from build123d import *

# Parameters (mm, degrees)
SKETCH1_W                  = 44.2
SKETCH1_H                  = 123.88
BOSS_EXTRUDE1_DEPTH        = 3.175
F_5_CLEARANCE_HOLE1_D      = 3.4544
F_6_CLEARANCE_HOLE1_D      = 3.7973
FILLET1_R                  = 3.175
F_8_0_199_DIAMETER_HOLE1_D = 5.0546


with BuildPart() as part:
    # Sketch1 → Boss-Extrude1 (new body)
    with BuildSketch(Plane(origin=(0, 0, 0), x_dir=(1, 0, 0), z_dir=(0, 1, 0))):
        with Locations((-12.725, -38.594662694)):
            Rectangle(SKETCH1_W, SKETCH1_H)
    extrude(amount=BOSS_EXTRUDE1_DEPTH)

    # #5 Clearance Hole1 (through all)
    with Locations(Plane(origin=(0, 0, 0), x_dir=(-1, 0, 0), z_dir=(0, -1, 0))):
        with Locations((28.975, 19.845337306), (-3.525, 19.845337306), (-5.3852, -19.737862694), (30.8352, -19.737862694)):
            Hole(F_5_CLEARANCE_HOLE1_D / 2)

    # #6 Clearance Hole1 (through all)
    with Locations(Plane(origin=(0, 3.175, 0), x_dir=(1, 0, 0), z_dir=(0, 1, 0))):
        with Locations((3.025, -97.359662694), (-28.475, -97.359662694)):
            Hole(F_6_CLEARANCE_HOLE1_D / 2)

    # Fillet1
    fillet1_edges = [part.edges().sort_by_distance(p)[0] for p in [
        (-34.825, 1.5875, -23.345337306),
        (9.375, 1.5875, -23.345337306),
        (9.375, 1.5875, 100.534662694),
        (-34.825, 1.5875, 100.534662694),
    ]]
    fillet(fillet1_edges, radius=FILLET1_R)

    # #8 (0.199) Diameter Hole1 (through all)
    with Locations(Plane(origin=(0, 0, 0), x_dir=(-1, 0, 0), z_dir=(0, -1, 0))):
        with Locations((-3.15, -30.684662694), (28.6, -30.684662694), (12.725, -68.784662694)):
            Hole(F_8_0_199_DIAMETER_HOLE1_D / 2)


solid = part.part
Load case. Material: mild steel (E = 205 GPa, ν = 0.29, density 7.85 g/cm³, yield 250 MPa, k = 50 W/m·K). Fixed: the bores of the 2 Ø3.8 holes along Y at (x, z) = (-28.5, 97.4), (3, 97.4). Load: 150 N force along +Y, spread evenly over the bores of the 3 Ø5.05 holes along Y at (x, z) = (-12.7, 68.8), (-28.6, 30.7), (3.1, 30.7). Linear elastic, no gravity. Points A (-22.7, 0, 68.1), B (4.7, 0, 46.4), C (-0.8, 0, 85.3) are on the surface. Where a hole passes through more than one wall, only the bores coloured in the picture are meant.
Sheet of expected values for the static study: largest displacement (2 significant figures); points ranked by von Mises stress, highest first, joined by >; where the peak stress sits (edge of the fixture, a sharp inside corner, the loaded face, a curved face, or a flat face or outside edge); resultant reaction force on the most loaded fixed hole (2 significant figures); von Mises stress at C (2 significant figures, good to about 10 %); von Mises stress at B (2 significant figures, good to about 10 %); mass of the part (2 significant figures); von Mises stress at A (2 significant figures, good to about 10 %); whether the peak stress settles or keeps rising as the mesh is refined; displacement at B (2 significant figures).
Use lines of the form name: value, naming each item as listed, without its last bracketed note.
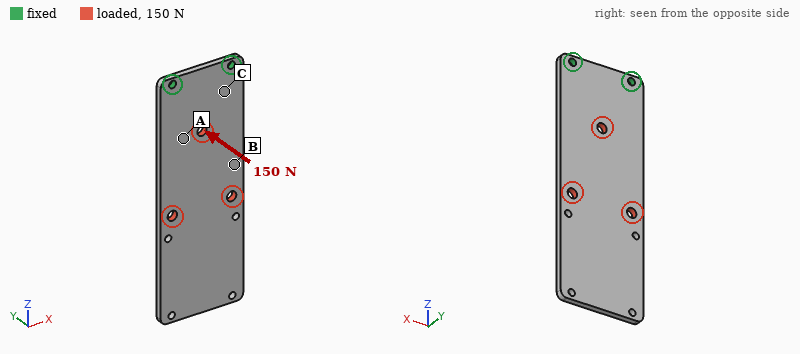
largest displacement: 1.1 mm
points ranked by von Mises stress, highest first, joined by >: C > A > B
where the peak stress sits: edge of the fixture
resultant reaction force on the most loaded fixed hole: 75 N
von Mises stress at C: 79 MPa
von Mises stress at B: 23 MPa
mass of the part: 130 g
von Mises stress at A: 55 MPa
whether the peak stress settles or keeps rising as the mesh is refined: keeps rising
displacement at B: 0.33 mm
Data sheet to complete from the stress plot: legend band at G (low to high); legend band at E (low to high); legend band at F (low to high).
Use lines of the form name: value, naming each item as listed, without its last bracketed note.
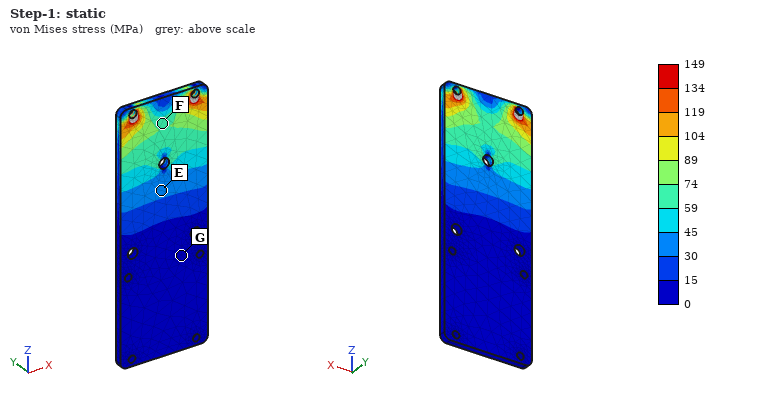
legend band at G: 0 to 15 MPa
legend band at E: 30 to 45 MPa
legend band at F: 59 to 74 MPa
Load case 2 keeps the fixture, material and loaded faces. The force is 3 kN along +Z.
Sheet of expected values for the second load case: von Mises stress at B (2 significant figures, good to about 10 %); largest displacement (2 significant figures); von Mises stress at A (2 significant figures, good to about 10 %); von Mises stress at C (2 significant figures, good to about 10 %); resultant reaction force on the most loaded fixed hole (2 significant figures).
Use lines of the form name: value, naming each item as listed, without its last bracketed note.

von Mises stress at B: 17 MPa
largest displacement: 7.5 µm
von Mises stress at A: 18 MPa
von Mises stress at C: 27 MPa
resultant reaction force on the most loaded fixed hole: 1.5 kN
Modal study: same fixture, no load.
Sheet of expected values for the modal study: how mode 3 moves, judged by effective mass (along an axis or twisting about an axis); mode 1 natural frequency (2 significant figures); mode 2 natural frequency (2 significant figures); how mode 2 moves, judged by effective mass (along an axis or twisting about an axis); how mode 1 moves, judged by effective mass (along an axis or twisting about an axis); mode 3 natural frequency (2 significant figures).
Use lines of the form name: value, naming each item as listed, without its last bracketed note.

how mode 3 moves, judged by effective mass: along Y
mode 1 natural frequency: 180 Hz
mode 2 natural frequency: 1000 Hz
how mode 2 moves, judged by effective mass: twisting about Z
how mode 1 moves, judged by effective mass: along Y
mode 3 natural frequency: 1100 Hz
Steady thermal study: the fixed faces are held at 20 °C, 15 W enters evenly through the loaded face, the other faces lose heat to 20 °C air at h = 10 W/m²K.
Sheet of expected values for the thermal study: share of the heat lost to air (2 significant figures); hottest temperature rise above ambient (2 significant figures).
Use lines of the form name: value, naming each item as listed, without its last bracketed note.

share of the heat lost to air: 40 %
hottest temperature rise above ambient: 79 K
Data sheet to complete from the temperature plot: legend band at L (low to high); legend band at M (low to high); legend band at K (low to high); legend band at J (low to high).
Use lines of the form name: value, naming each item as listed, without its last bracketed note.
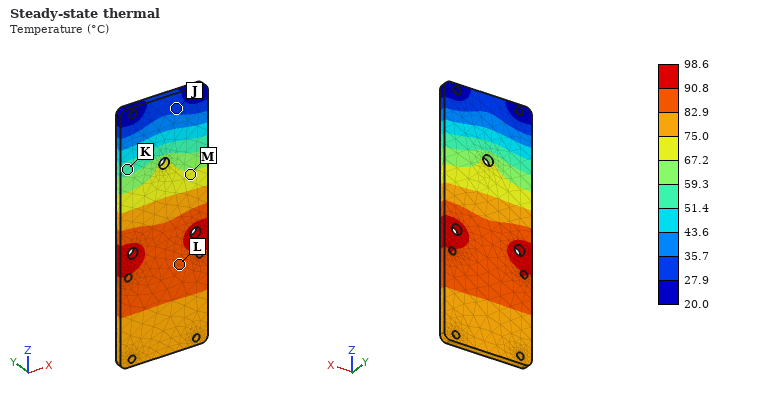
legend band at L: 82.9 to 90.8 °C
legend band at M: 67.2 to 75.0 °C
legend band at K: 51.4 to 59.3 °C
legend band at J: 27.9 to 35.7 °C
